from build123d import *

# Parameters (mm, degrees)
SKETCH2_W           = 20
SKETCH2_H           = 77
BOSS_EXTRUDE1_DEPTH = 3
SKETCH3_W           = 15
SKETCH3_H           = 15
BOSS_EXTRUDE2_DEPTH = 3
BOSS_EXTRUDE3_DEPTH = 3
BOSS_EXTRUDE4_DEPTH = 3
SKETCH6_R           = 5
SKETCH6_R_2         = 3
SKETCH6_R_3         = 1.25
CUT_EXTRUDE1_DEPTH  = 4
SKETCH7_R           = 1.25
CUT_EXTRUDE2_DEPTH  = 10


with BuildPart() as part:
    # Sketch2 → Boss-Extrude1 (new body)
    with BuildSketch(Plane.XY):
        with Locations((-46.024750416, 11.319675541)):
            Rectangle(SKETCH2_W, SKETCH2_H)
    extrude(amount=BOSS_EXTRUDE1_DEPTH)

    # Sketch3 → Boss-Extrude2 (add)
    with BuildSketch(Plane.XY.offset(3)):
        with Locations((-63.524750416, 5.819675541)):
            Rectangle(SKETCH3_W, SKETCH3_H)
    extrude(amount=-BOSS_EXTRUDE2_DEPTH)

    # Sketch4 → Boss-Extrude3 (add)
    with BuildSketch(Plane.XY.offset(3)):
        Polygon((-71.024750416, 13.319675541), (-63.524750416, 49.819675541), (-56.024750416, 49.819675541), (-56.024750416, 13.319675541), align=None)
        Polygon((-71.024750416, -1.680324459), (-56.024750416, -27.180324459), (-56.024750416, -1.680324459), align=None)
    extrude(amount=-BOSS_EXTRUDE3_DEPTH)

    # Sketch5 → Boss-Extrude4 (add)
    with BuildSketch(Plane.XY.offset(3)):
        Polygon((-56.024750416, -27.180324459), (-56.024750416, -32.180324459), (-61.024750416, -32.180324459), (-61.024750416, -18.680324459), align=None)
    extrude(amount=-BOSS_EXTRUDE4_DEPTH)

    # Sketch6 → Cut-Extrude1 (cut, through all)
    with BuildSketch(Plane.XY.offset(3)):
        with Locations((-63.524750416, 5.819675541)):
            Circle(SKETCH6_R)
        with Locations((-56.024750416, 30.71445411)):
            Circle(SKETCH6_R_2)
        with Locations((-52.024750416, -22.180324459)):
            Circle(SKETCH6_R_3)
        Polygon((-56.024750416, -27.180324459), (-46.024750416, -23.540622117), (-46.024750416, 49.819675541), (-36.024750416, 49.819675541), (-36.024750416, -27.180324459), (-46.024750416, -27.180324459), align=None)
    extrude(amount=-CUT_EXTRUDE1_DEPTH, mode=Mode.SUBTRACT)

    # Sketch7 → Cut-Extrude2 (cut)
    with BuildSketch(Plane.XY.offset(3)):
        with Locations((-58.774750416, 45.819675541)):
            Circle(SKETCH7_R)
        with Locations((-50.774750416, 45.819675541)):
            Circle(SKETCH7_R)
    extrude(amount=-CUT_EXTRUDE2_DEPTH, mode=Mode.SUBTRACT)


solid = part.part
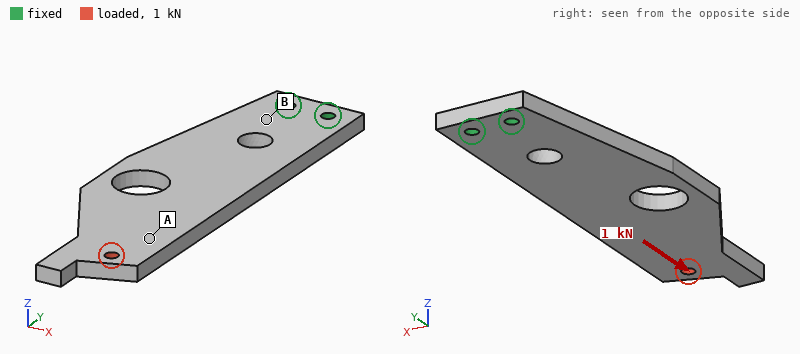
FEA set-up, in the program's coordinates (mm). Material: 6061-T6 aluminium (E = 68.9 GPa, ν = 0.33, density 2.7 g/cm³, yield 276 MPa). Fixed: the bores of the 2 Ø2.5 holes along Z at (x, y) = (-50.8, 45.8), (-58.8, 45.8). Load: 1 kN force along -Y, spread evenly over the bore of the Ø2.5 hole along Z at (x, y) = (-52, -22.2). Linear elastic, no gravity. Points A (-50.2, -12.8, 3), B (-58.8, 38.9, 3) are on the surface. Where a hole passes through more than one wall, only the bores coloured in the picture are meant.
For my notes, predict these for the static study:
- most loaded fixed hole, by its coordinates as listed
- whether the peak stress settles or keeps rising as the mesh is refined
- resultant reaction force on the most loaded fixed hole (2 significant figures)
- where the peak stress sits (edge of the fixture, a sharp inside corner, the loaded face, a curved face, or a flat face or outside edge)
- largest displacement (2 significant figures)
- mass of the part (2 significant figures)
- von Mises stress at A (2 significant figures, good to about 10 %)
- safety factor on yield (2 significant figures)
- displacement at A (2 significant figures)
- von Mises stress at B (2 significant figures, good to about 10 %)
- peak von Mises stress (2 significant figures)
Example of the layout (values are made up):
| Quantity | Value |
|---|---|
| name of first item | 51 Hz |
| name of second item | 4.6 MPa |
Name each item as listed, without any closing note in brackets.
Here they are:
| Quantity | Value |
|---|---|
| most loaded fixed hole, by its coordinates as listed | (-50.8, 45.8) |
| whether the peak stress settles or keeps rising as the mesh is refined | settles |
| resultant reaction force on the most loaded fixed hole | 790 N |
| where the peak stress sits | the loaded face |
| largest displacement | 90 µm |
| mass of the part | 12 g |
| von Mises stress at A | 30 MPa |
| safety factor on yield | 2.6 |
| displacement at A | 57 µm |
| von Mises stress at B | 11 MPa |
| peak von Mises stress | 110 MPa |
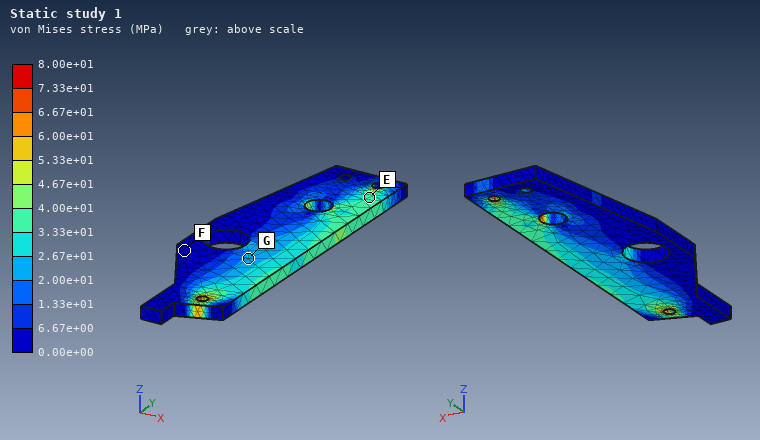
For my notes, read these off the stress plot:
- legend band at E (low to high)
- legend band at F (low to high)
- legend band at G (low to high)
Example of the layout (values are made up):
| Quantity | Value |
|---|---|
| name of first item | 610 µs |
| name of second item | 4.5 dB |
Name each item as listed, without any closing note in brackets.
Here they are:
| Quantity | Value |
|---|---|
| legend band at E | 3.33e+01 to 4.00e+01 MPa |
| legend band at F | 0.00e+00 to 6.67e+00 MPa |
| legend band at G | 2.00e+01 to 2.67e+01 MPa |
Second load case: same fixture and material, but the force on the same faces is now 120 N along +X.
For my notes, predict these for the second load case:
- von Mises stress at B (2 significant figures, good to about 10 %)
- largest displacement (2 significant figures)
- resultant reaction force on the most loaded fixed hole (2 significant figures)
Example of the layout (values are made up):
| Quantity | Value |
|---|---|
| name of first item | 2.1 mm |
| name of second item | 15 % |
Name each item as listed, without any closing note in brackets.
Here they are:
| Quantity | Value |
|---|---|
| von Mises stress at B | 18 MPa |
| largest displacement | 0.14 mm |
| resultant reaction force on the most loaded fixed hole | 830 N |
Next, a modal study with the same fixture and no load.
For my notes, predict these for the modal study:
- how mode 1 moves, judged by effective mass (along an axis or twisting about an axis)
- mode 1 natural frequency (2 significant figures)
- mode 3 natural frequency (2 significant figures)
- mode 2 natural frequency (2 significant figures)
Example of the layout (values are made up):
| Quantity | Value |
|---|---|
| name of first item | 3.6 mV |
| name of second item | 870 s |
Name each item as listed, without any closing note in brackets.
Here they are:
| Quantity | Value |
|---|---|
| how mode 1 moves, judged by effective mass | along Z |
| mode 1 natural frequency | 470 Hz |
| mode 3 natural frequency | 2600 Hz |
| mode 2 natural frequency | 2600 Hz |
